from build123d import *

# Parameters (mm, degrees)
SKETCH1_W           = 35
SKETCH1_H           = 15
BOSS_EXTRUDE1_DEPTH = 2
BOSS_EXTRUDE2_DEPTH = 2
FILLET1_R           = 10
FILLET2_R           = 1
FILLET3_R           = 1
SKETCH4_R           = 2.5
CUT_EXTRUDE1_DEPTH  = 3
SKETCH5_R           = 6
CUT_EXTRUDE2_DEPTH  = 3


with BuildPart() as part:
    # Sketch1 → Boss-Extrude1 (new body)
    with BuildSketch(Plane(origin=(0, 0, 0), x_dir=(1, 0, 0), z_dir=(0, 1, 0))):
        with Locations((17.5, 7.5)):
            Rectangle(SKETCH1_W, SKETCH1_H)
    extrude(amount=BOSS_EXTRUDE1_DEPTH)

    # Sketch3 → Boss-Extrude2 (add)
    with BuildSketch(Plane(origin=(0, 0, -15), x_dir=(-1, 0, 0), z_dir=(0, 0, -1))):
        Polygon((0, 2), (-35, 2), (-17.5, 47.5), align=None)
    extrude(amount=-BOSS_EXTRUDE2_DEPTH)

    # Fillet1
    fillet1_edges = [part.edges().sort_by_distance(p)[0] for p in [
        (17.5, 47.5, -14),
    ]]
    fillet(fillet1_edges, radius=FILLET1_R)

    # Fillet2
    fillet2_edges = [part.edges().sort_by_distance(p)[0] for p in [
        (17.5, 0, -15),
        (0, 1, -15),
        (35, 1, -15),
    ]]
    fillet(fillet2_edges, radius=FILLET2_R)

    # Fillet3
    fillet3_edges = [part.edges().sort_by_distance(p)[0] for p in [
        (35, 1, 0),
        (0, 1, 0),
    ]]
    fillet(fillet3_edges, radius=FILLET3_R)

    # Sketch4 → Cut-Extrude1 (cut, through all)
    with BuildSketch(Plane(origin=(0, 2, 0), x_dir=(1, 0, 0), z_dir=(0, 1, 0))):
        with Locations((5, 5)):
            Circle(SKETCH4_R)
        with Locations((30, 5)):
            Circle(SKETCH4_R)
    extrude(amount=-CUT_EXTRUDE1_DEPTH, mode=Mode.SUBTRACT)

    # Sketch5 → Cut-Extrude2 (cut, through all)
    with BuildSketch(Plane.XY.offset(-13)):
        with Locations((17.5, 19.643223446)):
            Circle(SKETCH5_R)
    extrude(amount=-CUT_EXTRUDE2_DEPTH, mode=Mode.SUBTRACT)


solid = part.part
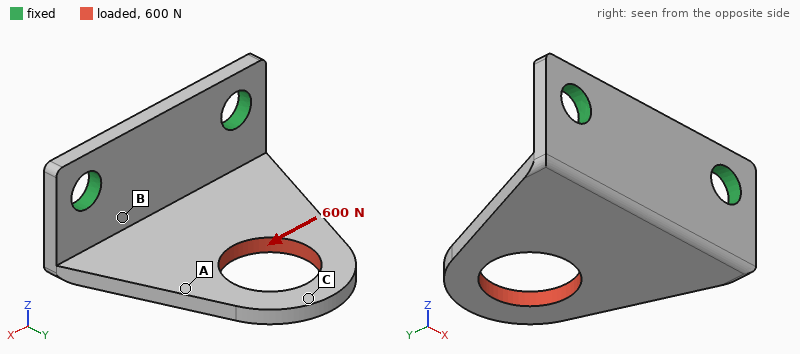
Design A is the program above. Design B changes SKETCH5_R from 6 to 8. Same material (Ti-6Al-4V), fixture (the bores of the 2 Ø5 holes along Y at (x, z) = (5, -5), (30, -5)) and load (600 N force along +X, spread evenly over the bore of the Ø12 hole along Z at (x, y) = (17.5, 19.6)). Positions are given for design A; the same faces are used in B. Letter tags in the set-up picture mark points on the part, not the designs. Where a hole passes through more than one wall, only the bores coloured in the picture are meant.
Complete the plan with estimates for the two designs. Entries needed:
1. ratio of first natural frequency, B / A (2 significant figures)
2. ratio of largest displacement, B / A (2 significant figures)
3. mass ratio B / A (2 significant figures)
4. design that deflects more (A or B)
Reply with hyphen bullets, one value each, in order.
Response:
- 1.2
- 1.4
- 0.91
- B
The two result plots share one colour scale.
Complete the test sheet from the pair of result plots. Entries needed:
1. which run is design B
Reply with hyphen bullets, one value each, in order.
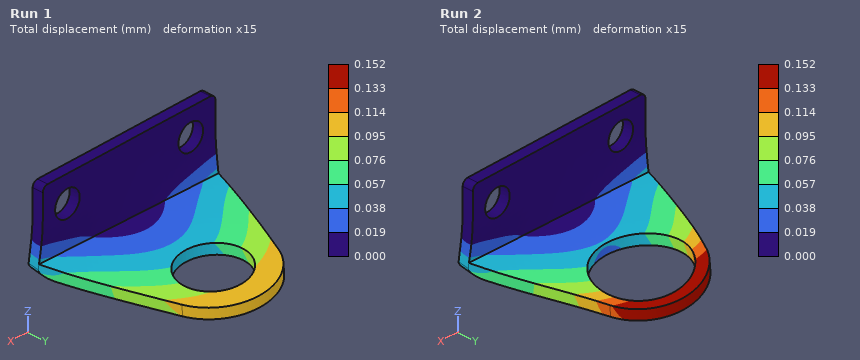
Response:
- Run 2
